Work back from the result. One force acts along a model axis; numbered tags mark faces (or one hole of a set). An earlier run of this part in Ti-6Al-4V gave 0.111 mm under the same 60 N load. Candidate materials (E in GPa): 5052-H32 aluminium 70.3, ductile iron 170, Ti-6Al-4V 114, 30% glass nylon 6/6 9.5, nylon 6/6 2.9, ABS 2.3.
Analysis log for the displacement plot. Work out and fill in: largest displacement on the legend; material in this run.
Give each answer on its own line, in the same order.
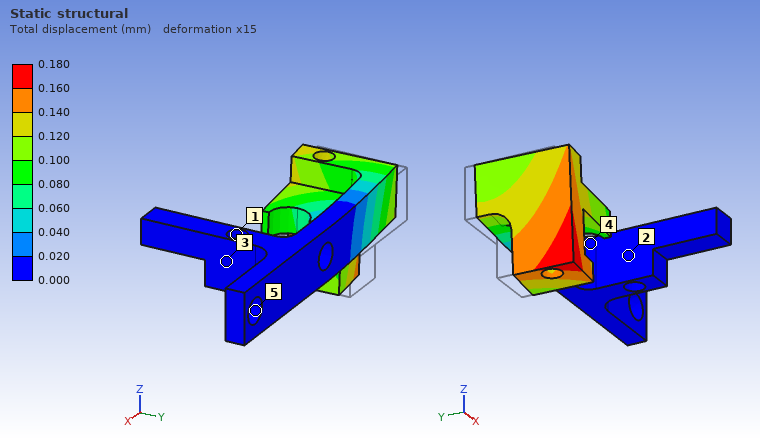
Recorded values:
0.180 mm
5052-H32 aluminium
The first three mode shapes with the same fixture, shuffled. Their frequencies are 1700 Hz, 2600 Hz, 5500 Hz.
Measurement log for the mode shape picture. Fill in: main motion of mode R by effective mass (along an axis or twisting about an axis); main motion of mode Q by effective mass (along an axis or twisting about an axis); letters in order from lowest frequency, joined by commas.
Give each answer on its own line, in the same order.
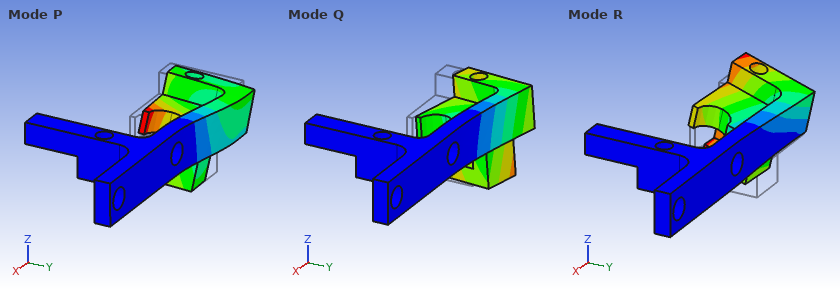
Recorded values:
along Z
along Y
Q, R, P
